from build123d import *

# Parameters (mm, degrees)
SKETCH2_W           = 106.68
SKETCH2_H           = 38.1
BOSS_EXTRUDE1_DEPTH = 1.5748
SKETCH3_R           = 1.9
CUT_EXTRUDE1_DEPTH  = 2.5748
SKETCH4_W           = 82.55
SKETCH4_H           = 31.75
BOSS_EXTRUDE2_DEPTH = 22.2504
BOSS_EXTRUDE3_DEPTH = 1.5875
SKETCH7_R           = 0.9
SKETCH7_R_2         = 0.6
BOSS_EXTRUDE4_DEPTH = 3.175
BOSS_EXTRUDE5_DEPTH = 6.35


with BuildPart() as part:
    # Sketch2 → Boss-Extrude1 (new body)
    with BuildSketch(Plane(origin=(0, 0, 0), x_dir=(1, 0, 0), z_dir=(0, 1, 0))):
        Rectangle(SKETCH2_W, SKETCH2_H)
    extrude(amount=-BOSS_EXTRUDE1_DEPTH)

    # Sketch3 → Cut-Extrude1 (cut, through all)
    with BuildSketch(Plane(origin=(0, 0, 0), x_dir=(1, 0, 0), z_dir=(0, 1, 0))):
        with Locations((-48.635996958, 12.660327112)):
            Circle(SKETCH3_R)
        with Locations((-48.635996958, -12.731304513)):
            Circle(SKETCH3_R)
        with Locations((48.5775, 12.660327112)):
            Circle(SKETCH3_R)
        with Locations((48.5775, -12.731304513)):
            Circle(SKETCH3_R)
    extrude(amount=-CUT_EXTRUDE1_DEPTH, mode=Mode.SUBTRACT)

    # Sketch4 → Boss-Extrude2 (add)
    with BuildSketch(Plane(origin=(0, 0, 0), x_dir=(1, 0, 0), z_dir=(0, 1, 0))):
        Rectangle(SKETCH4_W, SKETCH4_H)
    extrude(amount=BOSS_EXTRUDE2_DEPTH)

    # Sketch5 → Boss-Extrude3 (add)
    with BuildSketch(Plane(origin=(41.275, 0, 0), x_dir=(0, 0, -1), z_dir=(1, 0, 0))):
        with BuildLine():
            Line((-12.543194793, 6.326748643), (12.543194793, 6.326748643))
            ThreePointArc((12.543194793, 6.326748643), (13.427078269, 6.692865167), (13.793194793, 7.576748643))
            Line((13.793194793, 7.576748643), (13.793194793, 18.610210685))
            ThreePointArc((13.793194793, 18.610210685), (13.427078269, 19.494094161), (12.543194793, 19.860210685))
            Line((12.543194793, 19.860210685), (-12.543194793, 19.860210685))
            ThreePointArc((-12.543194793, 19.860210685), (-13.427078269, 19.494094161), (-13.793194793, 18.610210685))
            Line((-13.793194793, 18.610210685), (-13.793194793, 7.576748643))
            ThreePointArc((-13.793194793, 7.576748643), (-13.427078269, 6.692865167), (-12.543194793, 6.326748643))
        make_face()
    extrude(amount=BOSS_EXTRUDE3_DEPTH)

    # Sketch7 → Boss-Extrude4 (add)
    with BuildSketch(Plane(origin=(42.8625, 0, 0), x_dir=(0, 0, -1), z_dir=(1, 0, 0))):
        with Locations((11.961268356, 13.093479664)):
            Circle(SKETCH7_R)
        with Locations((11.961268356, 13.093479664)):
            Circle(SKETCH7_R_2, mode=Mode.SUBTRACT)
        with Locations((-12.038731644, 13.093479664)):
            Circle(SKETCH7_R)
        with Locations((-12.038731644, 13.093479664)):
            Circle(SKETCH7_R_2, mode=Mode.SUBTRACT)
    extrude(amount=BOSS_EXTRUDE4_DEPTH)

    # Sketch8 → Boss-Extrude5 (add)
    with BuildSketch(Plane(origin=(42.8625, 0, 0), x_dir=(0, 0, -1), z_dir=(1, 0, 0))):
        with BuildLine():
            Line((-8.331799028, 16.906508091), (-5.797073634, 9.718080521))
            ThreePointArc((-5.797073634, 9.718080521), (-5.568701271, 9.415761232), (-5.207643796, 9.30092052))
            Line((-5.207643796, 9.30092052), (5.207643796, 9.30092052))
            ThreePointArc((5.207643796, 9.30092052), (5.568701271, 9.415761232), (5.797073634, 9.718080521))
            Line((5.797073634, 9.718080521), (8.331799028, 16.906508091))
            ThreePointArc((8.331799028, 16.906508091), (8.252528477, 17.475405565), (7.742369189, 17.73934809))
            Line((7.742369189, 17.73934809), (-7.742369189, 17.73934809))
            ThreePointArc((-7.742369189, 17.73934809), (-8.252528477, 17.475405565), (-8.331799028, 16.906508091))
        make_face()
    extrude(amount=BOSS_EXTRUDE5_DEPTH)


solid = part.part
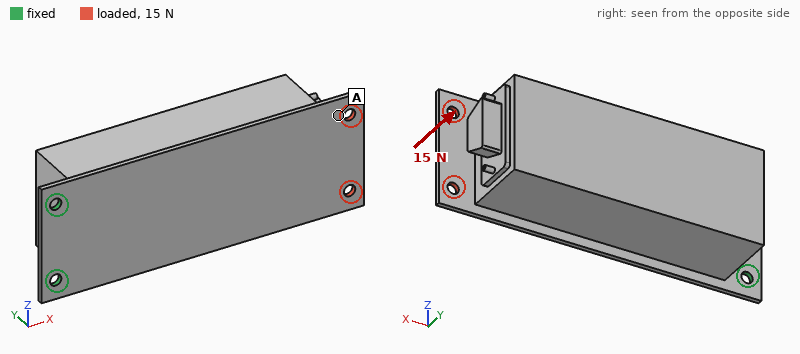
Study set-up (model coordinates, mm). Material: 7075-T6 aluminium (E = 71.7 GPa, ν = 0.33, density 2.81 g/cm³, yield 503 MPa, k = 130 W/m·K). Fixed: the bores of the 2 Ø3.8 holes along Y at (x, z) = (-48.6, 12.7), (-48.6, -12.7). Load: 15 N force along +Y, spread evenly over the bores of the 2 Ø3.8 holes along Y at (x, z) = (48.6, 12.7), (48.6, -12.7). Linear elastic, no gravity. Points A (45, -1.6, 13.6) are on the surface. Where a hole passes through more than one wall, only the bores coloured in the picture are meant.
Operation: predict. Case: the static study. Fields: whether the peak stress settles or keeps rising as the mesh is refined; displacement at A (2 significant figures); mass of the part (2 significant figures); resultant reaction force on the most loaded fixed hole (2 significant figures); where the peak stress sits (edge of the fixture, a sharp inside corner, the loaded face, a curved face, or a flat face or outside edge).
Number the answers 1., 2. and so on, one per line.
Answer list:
1. keeps rising
2. 1.0 mm
3. 190 g
4. 9.1 N
5. edge of the fixture
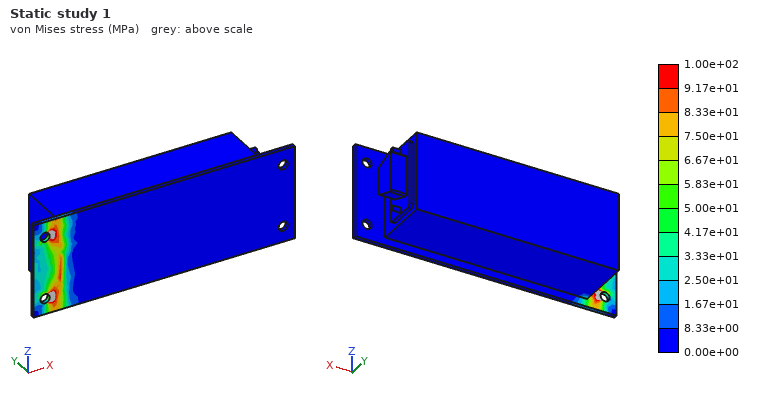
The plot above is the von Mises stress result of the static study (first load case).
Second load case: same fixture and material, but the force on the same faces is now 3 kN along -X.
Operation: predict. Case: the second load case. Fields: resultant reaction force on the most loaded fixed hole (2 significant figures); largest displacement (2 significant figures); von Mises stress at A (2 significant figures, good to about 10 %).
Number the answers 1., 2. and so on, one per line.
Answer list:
1. 1.5 kN
2. 0.16 mm
3. 99 MPa
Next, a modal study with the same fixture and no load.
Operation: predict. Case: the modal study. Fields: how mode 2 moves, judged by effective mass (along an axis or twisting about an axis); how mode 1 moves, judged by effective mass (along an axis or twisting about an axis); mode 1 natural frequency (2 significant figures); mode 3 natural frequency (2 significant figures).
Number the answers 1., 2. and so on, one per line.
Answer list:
1. along Z
2. along Y
3. 76 Hz
4. 1700 Hz
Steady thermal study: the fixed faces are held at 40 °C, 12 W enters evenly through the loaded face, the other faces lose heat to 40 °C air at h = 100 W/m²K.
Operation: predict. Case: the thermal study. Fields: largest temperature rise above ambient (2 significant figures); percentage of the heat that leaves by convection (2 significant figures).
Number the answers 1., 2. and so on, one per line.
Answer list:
1. 30 K
2. 78 %
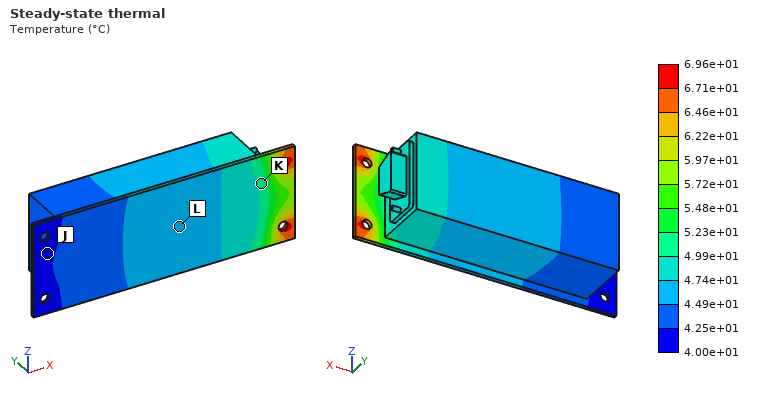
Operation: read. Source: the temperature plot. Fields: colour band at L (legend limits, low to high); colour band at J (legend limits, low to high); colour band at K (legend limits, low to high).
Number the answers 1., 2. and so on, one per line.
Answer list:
1. 4.49e+01 to 4.74e+01 °C
2. 4.00e+01 to 4.25e+01 °C
3. 4.99e+01 to 5.23e+01 °C
